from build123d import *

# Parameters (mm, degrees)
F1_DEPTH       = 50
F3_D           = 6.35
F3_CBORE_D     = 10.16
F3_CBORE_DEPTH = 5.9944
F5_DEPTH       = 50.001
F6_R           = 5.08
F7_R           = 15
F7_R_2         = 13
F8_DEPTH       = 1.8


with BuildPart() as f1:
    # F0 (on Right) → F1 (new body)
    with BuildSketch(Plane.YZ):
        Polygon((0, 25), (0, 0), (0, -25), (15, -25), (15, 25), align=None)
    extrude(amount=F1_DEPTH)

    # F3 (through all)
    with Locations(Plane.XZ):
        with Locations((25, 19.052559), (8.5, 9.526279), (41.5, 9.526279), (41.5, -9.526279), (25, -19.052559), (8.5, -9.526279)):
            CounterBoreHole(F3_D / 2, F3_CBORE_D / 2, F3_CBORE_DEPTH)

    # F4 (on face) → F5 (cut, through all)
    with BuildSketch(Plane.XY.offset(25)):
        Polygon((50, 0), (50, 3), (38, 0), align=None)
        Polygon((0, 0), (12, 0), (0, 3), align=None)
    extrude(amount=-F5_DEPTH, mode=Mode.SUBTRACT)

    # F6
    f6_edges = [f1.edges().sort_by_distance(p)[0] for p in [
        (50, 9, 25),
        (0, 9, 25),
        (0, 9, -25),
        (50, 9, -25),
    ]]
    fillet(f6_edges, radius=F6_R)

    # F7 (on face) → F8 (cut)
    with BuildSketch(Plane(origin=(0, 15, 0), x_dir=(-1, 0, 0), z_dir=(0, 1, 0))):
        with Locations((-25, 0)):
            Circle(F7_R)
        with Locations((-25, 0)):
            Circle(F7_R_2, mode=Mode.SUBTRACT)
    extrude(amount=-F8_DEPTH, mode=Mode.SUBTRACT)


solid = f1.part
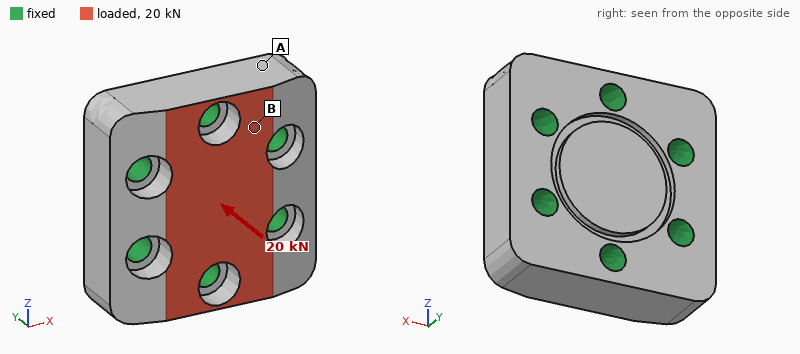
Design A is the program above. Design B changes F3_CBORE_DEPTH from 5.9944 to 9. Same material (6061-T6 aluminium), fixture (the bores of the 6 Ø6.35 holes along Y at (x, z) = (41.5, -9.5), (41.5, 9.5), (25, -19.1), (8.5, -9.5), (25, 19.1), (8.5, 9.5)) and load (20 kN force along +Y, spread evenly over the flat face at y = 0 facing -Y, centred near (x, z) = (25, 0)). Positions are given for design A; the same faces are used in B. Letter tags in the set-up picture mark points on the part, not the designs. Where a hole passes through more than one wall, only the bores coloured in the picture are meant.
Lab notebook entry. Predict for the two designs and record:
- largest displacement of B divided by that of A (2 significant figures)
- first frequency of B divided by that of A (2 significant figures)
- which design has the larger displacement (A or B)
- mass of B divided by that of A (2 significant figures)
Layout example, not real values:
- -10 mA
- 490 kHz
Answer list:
- 1.3
- 0.81
- B
- 0.97
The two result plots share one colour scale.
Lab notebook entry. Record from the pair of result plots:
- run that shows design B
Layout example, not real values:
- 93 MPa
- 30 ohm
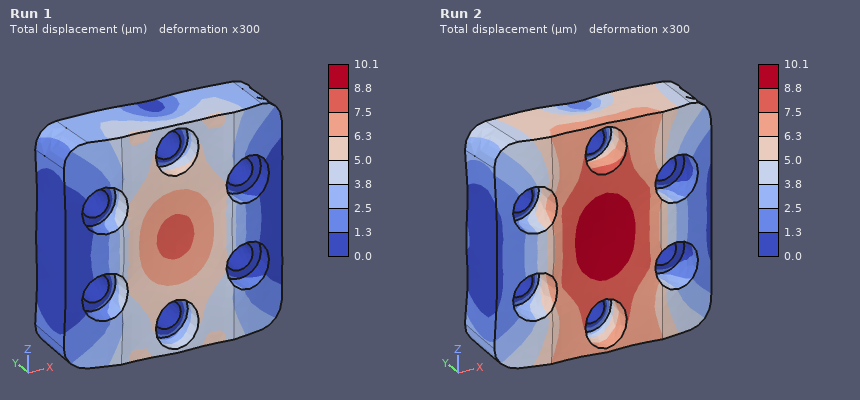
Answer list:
- Run 2
